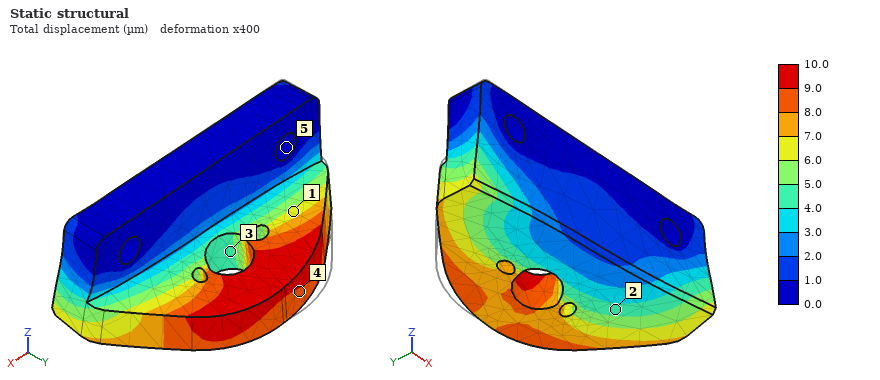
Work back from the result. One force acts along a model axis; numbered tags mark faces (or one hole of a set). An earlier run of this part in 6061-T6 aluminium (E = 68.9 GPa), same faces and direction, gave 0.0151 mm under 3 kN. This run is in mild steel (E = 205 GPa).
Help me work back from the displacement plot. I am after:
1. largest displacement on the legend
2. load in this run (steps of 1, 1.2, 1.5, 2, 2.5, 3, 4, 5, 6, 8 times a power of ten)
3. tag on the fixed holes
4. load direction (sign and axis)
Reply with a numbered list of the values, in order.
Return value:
1. 10.0 µm
2. 6 kN
3. 5
4. +X
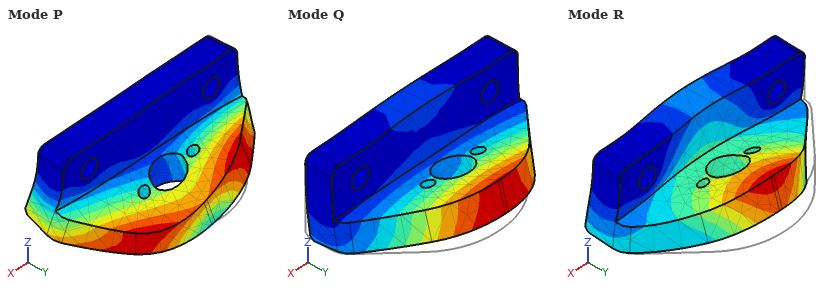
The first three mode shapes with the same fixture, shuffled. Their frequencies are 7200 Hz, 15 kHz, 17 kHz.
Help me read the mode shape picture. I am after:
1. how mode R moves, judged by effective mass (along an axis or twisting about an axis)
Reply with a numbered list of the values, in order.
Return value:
1. along Y
